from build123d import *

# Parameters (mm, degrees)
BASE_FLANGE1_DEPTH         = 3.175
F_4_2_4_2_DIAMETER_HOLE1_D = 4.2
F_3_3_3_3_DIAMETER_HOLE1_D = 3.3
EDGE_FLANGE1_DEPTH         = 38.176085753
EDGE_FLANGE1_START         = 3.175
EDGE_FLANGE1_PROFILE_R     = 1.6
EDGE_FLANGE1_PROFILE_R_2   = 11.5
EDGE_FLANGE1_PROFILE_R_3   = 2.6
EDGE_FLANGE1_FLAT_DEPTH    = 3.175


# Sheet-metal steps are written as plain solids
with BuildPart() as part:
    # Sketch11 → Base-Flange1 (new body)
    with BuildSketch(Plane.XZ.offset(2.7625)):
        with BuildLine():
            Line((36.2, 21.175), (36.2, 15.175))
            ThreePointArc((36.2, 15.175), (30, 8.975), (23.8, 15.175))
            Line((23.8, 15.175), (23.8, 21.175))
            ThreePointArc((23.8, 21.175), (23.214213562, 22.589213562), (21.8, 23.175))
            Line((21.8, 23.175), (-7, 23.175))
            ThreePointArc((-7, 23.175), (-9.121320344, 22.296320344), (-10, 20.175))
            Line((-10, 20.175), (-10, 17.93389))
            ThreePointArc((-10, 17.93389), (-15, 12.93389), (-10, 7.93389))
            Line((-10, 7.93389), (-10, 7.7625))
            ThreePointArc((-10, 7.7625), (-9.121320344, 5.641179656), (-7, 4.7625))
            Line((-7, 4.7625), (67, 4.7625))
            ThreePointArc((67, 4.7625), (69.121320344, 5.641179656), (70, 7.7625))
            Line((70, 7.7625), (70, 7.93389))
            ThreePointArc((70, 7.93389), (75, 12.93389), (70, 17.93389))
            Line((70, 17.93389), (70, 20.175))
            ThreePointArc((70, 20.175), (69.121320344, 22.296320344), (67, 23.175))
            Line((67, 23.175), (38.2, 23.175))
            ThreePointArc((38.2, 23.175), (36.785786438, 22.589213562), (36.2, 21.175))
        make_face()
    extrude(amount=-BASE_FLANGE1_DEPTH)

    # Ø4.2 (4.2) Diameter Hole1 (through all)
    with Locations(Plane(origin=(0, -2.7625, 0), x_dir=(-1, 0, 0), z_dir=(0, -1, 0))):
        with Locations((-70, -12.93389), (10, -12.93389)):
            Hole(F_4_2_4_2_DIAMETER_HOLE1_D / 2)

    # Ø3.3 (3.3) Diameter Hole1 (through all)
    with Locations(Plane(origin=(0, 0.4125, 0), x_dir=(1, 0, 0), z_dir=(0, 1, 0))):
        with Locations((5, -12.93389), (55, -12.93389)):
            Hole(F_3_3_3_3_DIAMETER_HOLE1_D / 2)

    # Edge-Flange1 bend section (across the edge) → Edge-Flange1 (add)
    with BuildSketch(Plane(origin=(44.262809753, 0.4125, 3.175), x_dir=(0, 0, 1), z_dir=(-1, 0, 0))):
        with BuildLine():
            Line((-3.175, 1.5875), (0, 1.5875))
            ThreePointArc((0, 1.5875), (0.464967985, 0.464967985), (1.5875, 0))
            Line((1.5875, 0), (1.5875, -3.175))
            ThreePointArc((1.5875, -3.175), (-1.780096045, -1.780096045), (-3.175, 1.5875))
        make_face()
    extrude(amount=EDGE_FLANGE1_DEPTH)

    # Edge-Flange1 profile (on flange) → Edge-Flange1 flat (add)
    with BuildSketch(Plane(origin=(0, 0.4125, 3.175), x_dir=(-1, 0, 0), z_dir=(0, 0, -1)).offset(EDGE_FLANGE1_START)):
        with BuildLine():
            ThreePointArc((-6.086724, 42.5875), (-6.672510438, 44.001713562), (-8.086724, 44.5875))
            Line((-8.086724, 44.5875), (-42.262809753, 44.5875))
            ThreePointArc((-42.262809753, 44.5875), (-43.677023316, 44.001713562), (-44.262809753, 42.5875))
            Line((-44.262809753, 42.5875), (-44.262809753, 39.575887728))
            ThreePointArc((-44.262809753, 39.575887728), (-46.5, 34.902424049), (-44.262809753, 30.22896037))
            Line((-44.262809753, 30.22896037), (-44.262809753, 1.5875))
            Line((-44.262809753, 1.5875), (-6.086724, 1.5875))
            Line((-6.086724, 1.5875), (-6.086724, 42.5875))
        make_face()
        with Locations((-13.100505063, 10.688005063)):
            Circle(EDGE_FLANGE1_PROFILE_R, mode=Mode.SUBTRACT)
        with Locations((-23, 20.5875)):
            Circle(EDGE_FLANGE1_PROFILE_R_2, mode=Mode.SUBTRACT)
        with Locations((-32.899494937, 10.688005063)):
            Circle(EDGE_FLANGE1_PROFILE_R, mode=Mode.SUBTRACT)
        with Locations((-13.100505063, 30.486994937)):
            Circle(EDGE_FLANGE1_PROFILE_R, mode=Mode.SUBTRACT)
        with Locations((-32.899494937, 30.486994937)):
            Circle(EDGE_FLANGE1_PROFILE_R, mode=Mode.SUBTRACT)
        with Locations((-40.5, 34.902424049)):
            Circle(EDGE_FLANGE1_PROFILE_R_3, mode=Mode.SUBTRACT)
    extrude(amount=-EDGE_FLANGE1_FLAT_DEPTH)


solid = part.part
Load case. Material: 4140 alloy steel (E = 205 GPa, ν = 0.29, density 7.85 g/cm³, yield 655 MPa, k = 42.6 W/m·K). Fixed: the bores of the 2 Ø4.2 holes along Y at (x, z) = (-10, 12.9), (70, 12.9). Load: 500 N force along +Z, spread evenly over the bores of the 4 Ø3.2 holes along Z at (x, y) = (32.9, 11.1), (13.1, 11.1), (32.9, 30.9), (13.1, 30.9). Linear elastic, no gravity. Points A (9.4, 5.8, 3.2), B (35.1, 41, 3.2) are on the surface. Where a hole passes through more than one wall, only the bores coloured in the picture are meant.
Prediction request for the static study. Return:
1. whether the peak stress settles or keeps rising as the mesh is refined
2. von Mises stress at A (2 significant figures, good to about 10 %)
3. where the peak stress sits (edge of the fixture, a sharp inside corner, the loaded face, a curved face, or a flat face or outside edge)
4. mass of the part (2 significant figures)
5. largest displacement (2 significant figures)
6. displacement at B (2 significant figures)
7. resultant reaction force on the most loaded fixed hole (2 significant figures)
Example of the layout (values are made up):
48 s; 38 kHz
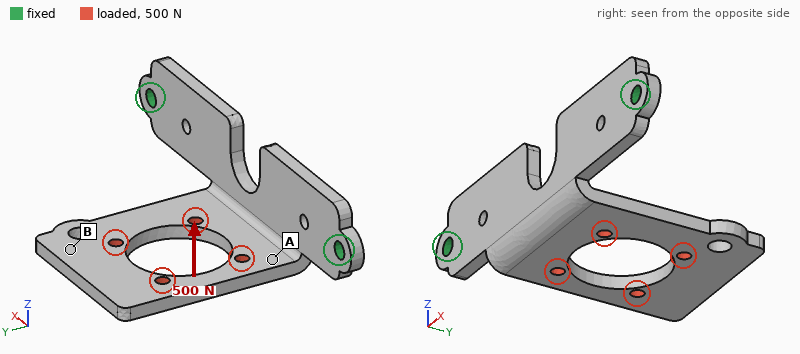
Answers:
keeps rising; 160 MPa; a sharp inside corner; 68 g; 1.1 mm; 0.95 mm; 500 N
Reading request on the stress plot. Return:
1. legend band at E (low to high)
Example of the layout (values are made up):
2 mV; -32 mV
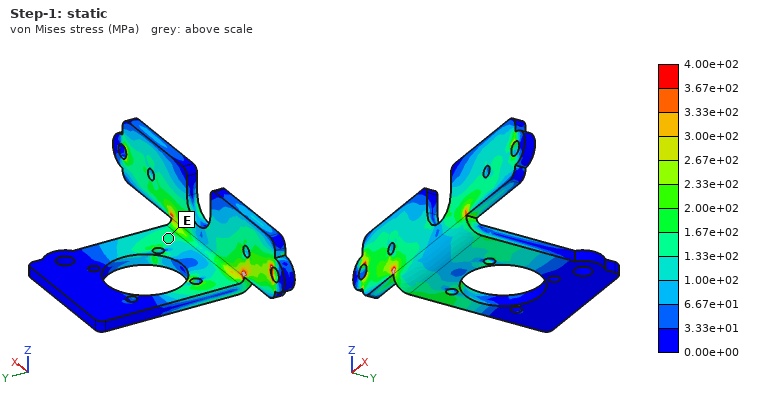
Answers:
1.33e+02 to 1.67e+02 MPa
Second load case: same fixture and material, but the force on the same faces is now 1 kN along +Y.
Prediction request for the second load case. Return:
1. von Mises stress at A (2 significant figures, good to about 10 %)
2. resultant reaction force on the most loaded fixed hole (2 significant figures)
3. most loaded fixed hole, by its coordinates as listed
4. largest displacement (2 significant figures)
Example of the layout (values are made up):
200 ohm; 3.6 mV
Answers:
59 MPa; 600 N; (-10, 12.9); 0.54 mm
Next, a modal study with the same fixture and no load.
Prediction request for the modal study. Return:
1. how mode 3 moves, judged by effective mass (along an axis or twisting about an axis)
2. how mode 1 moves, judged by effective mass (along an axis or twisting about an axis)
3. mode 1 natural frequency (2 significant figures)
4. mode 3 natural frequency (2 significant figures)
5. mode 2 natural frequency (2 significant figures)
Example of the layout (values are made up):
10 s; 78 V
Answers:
along Y; along Z; 660 Hz; 2200 Hz; 1600 Hz
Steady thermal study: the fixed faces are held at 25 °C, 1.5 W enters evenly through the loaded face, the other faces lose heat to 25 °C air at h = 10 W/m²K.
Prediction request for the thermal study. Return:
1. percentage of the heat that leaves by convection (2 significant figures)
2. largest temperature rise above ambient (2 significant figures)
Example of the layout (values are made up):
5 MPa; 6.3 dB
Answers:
35 %; 16 K
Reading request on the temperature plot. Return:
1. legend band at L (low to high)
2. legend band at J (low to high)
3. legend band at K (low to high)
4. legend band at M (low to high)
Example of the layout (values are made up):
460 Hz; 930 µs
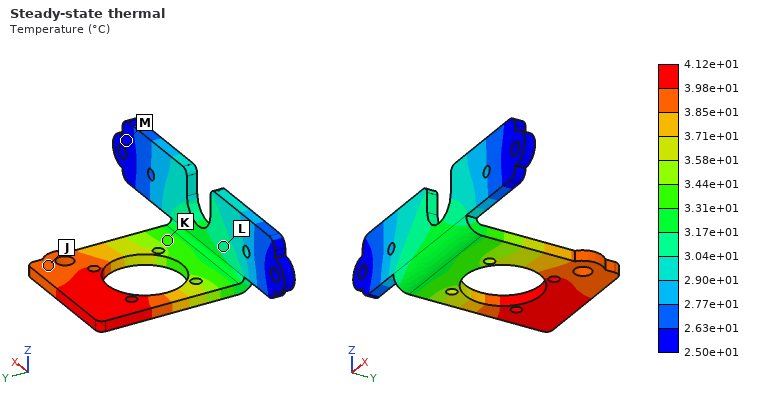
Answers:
3.04e+01 to 3.17e+01 °C; 3.85e+01 to 3.98e+01 °C; 3.31e+01 to 3.44e+01 °C; 2.50e+01 to 2.63e+01 °C
